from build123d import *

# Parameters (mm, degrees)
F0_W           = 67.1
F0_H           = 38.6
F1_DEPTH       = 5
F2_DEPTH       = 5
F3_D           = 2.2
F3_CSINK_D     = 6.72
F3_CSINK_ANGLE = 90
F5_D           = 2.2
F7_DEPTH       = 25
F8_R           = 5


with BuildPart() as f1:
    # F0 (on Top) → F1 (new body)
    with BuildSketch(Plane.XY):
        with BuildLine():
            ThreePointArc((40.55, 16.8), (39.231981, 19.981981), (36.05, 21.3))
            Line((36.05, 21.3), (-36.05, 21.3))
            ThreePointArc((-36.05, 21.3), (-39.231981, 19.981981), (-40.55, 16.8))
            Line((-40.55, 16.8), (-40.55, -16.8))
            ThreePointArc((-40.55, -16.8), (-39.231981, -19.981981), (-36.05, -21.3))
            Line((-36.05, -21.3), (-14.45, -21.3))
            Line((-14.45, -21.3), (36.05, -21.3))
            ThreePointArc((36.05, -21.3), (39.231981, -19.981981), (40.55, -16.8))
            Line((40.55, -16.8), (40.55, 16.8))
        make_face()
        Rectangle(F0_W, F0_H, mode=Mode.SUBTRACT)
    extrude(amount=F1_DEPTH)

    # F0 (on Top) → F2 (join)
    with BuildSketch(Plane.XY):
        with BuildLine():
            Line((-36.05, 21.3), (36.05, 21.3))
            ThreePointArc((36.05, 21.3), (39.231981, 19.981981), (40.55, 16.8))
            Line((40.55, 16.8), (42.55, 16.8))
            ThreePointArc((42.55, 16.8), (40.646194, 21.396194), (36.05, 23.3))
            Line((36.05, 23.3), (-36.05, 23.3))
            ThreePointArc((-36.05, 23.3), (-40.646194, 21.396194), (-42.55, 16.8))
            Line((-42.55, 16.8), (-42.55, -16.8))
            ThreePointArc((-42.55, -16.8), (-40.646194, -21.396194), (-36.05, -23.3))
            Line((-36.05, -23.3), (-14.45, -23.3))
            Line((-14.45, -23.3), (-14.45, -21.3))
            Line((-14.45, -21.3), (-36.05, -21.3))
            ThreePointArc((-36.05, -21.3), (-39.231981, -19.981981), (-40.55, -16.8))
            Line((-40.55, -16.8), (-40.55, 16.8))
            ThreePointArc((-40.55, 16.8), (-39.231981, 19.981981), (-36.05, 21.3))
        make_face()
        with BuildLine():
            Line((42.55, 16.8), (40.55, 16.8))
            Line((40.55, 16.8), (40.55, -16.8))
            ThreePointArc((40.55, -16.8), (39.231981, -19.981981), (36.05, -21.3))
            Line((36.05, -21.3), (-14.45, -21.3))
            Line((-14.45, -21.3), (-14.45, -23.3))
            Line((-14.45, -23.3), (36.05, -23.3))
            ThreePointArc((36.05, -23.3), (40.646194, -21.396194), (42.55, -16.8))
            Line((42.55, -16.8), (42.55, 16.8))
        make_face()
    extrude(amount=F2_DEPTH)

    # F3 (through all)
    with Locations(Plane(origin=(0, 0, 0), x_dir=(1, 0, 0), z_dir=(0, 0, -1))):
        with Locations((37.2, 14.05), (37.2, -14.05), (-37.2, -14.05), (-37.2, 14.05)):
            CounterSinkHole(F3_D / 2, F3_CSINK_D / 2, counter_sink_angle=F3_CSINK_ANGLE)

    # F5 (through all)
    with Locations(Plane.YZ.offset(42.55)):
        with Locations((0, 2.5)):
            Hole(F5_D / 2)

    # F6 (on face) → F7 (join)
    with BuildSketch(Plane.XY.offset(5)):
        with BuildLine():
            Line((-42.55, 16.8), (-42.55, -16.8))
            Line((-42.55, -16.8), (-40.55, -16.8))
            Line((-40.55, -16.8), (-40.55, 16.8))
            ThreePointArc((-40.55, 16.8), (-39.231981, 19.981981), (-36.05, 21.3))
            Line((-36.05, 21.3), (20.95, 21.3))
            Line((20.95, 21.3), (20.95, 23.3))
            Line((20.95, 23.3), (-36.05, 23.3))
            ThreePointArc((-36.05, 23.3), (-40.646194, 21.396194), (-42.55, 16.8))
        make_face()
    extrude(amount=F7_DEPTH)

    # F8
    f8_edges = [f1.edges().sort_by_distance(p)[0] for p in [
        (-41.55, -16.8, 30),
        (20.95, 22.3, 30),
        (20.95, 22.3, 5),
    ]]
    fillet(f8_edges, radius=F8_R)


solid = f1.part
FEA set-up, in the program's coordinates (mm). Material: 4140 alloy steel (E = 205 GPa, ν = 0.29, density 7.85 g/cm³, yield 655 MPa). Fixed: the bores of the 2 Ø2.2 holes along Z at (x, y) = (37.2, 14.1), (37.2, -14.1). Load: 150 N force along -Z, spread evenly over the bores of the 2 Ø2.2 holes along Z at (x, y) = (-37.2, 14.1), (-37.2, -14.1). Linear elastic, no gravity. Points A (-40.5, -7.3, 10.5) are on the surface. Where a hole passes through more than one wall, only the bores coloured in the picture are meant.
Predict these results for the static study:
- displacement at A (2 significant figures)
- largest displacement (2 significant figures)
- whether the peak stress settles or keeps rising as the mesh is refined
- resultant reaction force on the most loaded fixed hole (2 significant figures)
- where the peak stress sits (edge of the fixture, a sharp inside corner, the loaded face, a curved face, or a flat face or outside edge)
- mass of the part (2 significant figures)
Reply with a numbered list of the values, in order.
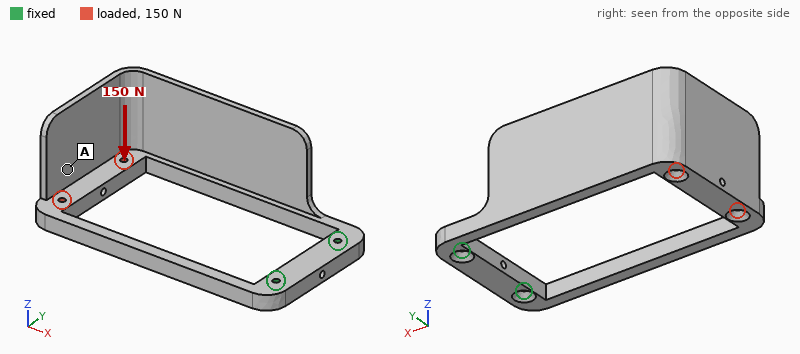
1. 1.1 mm
2. 1.2 mm
3. keeps rising
4. 82 N
5. edge of the fixture
6. 89 g
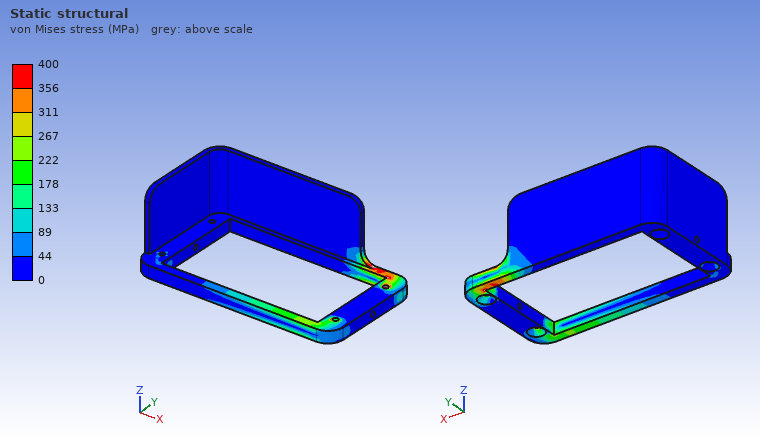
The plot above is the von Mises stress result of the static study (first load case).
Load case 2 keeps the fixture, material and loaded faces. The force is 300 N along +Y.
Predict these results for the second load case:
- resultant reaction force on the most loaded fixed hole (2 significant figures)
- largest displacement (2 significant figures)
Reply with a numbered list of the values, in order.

1. 670 N
2. 0.84 mm
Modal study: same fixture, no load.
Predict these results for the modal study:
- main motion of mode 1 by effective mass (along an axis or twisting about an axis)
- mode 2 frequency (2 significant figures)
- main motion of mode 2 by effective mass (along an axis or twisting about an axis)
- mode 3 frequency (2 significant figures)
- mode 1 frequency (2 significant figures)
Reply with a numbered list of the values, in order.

1. along Z
2. 410 Hz
3. along Y
4. 770 Hz
5. 270 Hz
